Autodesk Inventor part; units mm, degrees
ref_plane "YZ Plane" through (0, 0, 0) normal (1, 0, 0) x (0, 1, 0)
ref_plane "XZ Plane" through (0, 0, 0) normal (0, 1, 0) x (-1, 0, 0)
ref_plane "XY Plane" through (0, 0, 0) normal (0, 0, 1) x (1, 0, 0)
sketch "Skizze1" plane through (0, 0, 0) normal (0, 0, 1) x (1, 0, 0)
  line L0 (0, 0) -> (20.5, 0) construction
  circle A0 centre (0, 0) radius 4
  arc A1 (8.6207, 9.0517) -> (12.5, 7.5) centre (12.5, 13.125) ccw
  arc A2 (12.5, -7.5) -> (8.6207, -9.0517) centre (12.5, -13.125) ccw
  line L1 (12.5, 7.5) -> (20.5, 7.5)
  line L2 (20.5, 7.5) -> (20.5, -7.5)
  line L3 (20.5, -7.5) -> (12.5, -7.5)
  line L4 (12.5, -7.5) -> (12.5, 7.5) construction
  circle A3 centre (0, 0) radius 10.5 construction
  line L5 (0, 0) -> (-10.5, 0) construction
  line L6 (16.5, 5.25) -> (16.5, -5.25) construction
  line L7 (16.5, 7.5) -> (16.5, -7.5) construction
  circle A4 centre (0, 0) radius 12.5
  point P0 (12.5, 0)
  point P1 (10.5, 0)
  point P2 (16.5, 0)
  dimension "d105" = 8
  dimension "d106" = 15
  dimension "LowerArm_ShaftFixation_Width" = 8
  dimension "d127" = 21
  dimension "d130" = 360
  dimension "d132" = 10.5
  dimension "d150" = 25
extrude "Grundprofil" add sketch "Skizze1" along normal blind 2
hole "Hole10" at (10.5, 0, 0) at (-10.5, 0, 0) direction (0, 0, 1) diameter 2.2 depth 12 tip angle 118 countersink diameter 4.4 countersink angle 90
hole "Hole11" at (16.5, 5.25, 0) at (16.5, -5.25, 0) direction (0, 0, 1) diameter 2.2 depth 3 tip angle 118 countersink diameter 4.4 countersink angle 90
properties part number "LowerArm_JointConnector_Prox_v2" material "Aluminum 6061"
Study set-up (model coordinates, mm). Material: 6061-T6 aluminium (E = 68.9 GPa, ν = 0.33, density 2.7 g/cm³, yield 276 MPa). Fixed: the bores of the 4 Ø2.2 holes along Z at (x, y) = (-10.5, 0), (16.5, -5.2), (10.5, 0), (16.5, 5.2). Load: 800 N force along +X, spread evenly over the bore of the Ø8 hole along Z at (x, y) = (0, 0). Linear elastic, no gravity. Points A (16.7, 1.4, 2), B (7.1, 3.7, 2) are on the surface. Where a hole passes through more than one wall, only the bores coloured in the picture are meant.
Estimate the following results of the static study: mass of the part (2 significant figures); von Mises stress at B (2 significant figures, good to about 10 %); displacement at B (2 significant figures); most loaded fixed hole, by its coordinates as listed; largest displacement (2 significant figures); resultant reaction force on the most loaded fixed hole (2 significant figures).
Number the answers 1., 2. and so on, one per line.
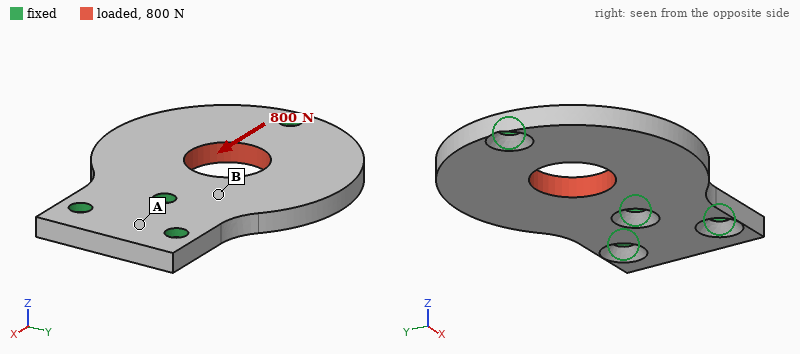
1. 3.0 g
2. 20 MPa
3. 1.9 µm
4. (-10.5, 0)
5. 3.9 µm
6. 320 N
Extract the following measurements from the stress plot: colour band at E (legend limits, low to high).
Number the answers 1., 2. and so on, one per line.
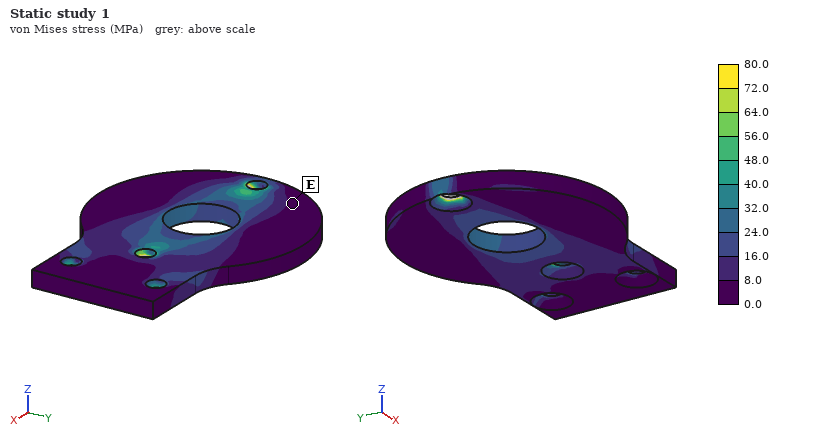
1. 0.0 to 8.0 MPa
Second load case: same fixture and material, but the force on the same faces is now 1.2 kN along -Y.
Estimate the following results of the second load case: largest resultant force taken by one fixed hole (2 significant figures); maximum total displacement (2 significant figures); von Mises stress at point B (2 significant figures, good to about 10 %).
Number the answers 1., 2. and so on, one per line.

1. 580 N
2. 20 µm
3. 25 MPa
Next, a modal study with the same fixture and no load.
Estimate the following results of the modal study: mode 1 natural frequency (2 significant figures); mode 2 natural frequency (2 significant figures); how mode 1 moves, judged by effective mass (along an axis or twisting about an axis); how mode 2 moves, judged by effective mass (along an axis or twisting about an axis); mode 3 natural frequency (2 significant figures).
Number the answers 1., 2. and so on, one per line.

1. 7800 Hz
2. 10 kHz
3. twisting about X
4. along Z
5. 24 kHz
